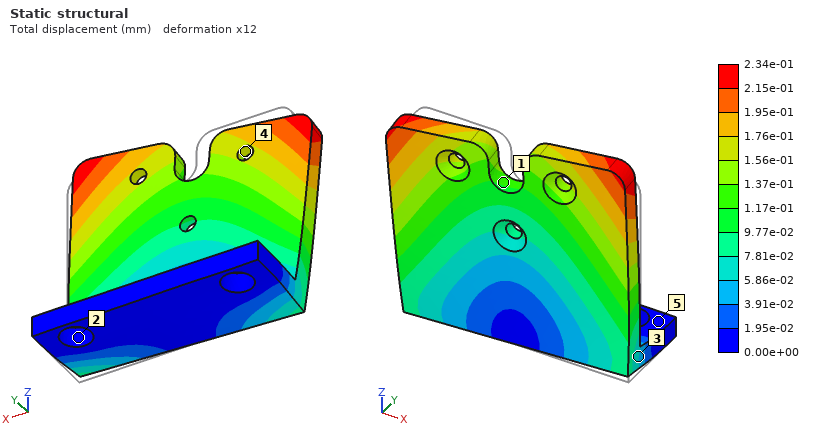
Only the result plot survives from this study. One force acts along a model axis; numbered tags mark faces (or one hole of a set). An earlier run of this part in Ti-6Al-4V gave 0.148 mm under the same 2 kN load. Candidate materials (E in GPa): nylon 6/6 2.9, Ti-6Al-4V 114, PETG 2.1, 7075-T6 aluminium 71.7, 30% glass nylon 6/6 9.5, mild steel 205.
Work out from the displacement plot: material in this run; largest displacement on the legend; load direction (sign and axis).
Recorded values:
7075-T6 aluminium
2.34e-01 mm
-X
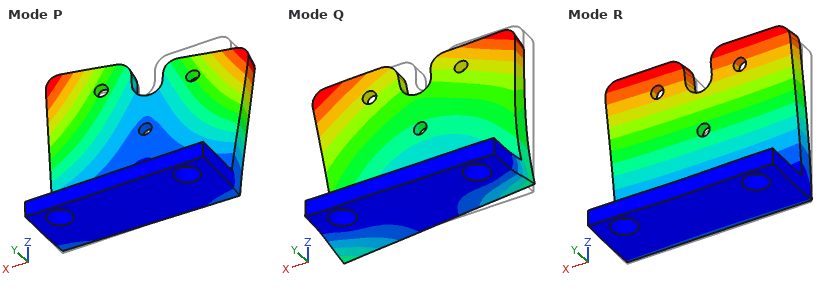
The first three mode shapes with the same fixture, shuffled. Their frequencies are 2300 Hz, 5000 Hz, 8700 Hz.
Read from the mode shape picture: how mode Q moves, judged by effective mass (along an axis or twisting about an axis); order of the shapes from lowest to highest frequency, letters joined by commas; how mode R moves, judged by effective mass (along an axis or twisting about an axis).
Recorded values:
along X
R, P, Q
along Y
